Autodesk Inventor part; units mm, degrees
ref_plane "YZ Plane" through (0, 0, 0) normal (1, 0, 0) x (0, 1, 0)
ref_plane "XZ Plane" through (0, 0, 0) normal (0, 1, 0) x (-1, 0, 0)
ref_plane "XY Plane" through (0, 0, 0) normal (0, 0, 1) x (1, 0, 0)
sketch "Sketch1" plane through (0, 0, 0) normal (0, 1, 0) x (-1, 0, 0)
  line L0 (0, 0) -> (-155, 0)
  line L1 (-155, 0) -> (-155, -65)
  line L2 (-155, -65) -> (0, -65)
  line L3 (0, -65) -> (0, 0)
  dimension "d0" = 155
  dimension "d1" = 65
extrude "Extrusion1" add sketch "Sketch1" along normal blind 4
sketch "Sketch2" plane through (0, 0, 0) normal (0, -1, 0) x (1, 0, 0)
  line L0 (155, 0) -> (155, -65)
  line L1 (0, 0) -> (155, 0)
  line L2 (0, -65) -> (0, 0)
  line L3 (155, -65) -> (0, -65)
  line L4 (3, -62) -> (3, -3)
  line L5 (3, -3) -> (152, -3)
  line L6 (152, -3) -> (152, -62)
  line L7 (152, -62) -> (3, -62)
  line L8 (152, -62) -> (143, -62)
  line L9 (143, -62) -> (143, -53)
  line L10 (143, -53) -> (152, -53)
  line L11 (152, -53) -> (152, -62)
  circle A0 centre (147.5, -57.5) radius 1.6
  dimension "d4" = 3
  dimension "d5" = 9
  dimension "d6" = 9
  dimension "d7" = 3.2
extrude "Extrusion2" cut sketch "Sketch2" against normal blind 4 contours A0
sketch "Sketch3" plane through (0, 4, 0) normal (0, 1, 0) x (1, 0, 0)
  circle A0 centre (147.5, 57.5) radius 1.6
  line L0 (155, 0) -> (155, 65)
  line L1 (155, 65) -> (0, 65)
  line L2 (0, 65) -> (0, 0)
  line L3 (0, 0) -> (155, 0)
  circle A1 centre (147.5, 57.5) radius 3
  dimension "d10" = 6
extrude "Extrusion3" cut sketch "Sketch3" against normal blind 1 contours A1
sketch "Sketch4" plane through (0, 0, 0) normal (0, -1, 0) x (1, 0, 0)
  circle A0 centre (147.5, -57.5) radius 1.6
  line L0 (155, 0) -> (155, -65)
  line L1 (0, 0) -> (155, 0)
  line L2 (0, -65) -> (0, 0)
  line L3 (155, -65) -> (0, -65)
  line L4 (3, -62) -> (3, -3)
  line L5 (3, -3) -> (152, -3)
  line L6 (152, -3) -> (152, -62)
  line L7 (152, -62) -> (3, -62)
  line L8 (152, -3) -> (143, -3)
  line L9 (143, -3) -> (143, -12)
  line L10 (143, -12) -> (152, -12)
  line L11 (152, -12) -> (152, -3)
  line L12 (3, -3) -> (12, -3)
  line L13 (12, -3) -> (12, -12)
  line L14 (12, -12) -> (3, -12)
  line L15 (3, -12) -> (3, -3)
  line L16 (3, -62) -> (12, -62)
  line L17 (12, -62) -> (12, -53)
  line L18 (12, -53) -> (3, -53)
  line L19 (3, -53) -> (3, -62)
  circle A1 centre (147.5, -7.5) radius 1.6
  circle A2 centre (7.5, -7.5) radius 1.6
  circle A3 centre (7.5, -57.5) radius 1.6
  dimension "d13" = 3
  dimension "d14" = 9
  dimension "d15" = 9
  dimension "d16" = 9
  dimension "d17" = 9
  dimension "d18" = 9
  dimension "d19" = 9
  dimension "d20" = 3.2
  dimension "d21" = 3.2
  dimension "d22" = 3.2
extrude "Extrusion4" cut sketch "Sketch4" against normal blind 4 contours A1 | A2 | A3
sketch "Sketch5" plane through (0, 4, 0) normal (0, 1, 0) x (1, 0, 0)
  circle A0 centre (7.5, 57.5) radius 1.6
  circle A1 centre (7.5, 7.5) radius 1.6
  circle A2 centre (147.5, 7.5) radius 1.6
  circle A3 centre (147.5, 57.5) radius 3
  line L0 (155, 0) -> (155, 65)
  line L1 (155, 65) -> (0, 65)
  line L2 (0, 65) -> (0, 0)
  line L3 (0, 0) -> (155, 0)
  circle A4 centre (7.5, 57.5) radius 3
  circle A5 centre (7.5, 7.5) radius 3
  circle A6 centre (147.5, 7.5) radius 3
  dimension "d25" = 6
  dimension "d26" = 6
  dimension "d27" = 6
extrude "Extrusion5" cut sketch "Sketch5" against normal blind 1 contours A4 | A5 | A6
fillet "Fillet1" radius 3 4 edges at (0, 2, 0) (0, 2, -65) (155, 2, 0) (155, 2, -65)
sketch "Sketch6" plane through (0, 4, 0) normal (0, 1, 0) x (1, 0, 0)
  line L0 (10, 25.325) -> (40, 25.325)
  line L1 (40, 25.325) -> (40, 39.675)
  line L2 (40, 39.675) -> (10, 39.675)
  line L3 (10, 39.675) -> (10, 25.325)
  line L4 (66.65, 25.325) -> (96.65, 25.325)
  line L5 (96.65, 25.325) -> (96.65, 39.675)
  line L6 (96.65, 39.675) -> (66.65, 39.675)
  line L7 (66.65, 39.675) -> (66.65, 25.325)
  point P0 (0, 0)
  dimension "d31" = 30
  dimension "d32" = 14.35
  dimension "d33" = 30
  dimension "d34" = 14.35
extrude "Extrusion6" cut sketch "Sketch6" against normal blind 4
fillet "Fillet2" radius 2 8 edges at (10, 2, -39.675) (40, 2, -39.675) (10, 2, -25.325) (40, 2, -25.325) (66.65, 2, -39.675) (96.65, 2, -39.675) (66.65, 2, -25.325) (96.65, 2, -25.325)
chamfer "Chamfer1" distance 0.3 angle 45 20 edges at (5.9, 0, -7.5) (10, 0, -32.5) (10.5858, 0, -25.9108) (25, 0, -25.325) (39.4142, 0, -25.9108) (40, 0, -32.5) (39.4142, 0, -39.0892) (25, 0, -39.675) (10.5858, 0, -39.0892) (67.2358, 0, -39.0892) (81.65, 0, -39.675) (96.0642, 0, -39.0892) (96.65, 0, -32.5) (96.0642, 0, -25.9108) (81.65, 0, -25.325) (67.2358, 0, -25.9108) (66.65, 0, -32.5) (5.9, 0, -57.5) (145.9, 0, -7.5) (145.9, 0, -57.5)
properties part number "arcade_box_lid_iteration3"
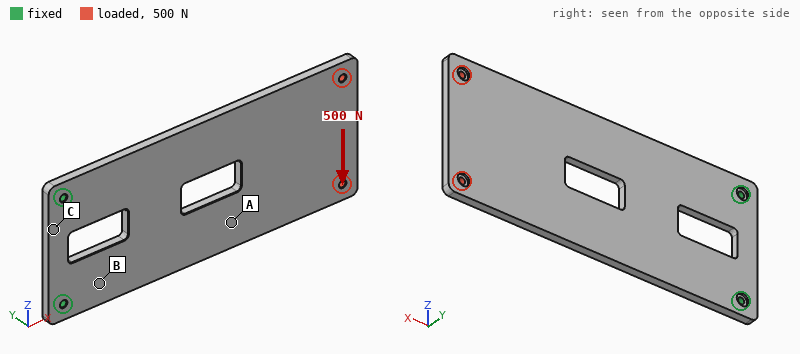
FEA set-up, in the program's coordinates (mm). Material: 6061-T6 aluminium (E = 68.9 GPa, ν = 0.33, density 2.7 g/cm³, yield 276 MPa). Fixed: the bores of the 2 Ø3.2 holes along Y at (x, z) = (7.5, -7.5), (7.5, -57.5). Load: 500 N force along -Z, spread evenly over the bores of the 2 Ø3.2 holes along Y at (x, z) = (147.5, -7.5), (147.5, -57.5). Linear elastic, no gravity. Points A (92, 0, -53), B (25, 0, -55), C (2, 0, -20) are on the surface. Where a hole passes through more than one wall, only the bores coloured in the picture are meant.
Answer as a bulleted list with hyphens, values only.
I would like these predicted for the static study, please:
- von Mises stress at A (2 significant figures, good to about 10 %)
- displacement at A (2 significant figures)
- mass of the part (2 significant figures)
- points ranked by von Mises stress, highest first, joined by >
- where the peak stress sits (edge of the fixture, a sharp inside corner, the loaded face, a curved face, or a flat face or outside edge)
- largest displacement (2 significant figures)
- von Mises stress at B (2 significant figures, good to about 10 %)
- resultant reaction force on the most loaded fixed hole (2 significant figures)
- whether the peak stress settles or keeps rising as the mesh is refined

- 8.6 MPa
- 0.061 mm
- 99 g
- B > A > C
- edge of the fixture
- 0.12 mm
- 18 MPa
- 1.4 kN
- keeps rising
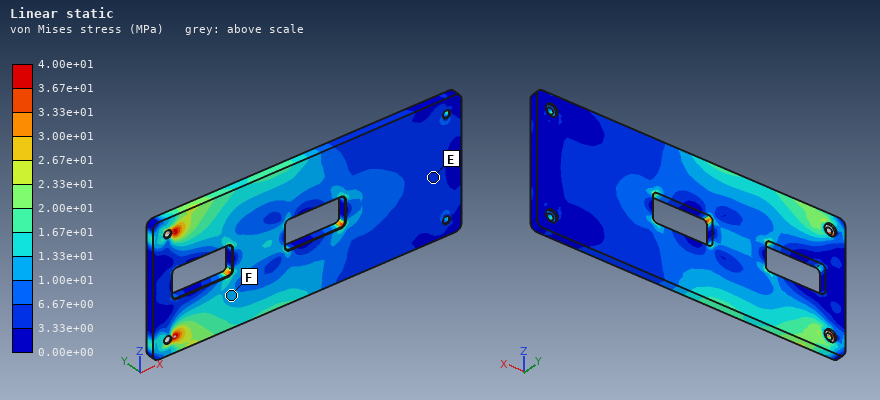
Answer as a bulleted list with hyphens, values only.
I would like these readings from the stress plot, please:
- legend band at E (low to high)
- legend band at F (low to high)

- 3.33e+00 to 6.67e+00 MPa
- 1.00e+01 to 1.33e+01 MPa
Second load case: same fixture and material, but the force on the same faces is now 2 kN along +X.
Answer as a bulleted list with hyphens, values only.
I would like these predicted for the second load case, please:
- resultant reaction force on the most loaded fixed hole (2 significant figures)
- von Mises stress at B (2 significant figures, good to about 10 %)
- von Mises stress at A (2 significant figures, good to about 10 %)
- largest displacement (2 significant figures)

- 1.0 kN
- 17 MPa
- 14 MPa
- 0.36 mm
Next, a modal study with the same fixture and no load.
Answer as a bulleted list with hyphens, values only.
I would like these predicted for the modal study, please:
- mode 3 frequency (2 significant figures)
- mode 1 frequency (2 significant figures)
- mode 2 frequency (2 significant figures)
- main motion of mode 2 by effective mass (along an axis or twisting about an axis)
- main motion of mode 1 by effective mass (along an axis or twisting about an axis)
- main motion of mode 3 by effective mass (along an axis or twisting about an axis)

- 840 Hz
- 130 Hz
- 650 Hz
- twisting about X
- along Y
- along Y
